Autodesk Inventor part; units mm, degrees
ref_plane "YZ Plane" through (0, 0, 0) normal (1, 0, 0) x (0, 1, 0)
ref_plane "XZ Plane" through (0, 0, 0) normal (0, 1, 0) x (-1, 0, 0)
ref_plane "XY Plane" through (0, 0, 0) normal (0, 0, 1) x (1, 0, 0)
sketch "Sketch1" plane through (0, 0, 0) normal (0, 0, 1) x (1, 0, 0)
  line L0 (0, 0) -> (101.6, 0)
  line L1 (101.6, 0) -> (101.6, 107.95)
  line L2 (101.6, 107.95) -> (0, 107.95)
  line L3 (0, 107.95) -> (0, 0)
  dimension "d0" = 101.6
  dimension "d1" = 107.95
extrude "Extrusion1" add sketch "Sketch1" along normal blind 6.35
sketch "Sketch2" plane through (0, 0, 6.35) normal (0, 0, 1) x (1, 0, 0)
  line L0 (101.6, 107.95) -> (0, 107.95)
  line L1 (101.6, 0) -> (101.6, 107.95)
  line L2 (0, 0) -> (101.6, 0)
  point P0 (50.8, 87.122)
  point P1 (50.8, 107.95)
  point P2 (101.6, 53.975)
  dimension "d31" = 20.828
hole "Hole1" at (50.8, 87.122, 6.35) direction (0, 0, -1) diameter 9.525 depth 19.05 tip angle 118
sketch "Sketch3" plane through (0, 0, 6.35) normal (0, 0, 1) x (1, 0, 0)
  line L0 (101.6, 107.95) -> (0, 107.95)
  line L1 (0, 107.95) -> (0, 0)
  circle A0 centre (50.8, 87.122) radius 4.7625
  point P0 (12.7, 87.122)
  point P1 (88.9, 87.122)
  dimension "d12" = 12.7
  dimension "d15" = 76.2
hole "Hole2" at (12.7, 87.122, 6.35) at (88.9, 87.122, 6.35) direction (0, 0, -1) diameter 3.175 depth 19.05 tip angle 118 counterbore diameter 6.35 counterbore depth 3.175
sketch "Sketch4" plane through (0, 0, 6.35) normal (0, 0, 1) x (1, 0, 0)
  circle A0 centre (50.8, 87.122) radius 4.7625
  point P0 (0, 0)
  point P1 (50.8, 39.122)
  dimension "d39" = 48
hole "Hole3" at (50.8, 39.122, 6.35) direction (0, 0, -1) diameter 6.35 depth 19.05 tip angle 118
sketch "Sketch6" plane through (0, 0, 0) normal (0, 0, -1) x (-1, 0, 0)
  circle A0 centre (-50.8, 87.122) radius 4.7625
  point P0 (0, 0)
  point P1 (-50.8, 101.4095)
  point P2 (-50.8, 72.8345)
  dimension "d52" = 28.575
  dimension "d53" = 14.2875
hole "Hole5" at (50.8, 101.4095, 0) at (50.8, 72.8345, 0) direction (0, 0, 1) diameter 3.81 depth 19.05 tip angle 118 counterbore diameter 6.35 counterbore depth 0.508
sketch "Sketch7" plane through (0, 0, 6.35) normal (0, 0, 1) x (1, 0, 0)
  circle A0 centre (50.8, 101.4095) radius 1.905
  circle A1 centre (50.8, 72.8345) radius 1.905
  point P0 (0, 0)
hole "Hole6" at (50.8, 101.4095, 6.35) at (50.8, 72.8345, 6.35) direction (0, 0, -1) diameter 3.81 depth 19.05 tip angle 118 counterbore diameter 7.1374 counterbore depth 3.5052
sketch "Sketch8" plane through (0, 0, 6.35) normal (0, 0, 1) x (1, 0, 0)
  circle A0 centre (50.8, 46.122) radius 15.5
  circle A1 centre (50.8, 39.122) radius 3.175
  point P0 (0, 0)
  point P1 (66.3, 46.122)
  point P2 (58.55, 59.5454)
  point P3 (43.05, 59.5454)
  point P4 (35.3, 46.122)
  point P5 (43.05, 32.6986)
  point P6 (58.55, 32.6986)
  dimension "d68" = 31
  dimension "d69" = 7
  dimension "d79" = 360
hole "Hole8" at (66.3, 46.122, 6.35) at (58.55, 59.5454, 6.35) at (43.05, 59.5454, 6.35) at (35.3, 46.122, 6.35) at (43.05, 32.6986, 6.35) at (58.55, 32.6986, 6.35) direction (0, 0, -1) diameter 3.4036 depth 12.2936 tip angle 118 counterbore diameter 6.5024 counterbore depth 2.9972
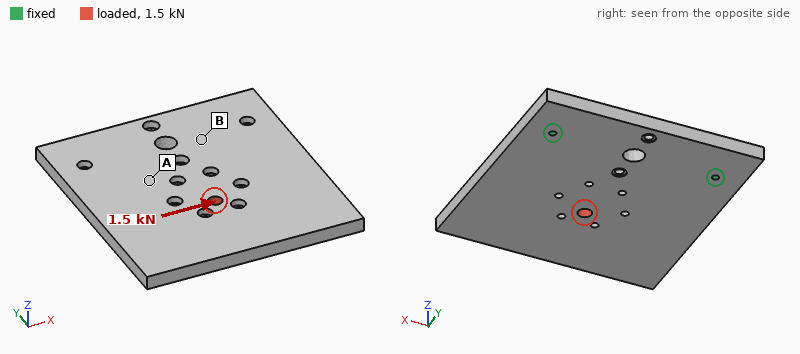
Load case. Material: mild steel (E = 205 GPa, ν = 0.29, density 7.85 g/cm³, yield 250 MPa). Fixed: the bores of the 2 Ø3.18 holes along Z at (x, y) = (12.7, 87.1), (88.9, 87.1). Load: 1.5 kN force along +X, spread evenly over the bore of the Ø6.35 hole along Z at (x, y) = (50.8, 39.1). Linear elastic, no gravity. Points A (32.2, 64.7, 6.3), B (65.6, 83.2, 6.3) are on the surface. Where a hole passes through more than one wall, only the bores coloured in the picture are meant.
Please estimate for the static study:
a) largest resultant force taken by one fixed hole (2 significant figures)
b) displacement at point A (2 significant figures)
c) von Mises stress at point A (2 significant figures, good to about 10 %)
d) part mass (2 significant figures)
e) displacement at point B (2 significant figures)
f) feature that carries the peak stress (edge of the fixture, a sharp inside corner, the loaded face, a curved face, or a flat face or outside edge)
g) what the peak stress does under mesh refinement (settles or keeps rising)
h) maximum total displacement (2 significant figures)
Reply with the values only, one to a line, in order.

1.2 kN
2.0 µm
4.7 MPa
530 g
0.95 µm
edge of the fixture
keeps rising
6.2 µm
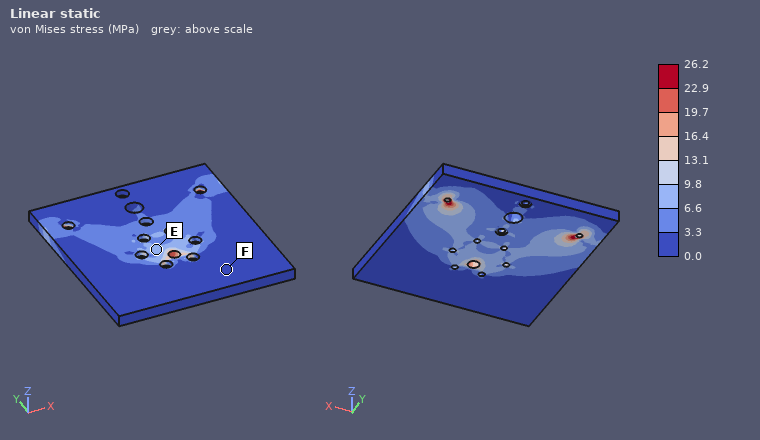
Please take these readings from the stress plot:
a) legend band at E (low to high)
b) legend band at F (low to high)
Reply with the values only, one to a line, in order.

6.6 to 9.8 MPa
0.0 to 3.3 MPa
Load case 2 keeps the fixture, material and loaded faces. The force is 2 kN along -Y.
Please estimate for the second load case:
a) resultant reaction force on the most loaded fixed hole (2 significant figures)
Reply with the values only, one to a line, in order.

1.0 kN
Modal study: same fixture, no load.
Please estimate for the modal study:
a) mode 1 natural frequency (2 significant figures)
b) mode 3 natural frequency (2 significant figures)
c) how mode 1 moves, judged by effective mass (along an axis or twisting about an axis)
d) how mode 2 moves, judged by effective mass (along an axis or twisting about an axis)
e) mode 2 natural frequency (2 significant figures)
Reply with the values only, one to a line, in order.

400 Hz
3100 Hz
along Z
twisting about Y
1300 Hz
